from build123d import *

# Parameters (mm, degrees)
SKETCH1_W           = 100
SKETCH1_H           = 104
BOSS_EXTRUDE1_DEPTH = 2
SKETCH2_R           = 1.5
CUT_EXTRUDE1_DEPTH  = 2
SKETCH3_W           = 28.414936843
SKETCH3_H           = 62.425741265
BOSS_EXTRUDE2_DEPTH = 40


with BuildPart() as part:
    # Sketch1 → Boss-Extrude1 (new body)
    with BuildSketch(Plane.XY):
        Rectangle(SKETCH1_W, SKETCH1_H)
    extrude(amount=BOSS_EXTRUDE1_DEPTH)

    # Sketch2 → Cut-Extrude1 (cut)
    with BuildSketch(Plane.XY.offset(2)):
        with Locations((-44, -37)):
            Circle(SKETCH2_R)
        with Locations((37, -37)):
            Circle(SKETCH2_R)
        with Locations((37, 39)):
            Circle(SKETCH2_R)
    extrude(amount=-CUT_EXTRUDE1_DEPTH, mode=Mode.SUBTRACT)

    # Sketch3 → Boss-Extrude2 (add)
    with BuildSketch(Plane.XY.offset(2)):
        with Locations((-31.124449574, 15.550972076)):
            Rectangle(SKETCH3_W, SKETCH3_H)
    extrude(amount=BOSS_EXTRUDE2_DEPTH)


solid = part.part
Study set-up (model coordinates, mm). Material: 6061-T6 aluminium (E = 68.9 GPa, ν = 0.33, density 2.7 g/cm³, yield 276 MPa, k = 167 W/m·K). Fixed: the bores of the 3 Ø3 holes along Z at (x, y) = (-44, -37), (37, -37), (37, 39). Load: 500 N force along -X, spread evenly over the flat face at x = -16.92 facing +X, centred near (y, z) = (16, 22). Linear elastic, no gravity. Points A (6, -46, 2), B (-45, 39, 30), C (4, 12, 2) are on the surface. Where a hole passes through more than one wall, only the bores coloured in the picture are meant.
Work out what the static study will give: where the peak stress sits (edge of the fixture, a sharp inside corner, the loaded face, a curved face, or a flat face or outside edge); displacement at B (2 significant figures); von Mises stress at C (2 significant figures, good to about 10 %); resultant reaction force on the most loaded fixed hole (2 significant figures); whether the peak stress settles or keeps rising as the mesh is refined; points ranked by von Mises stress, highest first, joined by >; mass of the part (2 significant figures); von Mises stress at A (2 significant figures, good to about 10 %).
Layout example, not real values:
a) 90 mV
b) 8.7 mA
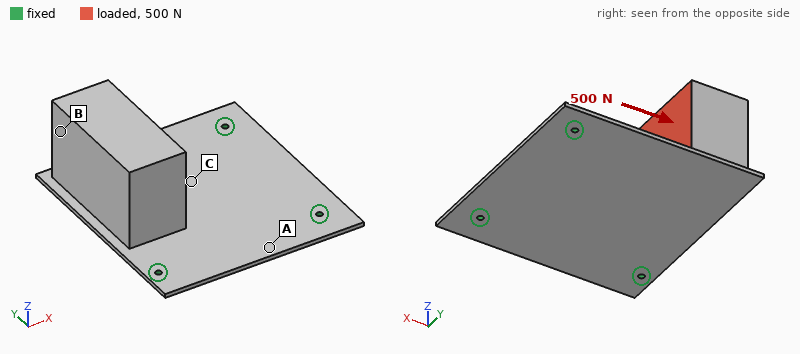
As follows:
a) edge of the fixture
b) 1.3 mm
c) 48 MPa
d) 220 N
e) keeps rising
f) C > A > B
g) 250 g
h) 26 MPa
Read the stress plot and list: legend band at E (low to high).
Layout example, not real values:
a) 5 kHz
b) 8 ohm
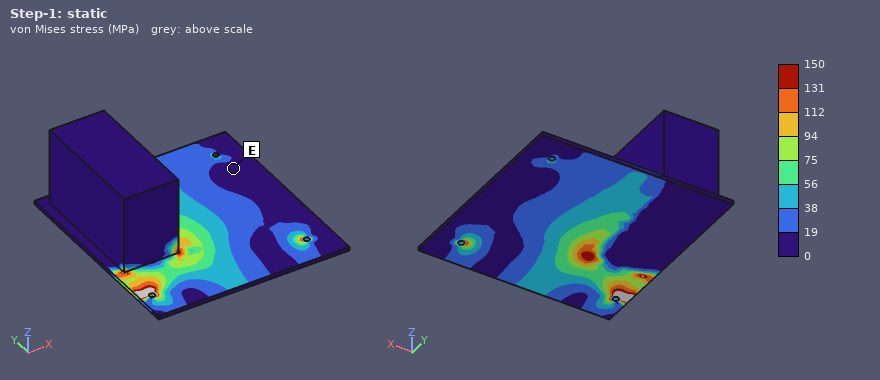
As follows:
a) 0 to 19 MPa
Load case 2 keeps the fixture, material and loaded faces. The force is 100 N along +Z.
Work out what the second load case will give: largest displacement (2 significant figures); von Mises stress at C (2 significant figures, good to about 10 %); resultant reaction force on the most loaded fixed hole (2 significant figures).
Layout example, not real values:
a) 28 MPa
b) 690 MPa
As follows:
a) 0.62 mm
b) 17 MPa
c) 58 N
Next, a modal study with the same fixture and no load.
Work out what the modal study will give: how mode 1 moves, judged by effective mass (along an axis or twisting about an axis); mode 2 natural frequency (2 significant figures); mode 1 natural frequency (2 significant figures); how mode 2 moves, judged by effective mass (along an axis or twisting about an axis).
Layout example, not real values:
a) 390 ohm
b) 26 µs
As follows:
a) along Z
b) 370 Hz
c) 140 Hz
d) along X
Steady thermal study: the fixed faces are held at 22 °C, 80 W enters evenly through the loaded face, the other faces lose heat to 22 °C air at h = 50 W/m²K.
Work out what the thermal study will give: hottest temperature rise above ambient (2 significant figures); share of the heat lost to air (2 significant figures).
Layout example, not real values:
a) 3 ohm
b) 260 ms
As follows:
a) 64 K
b) 59 %
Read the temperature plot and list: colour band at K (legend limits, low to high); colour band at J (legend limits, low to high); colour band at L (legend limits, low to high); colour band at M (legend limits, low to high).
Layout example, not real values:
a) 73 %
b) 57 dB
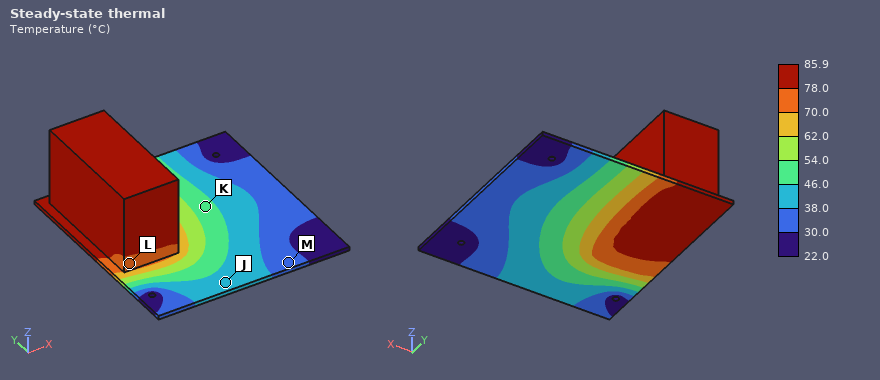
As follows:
a) 46.0 to 54.0 °C
b) 38.0 to 46.0 °C
c) 70.0 to 78.0 °C
d) 30.0 to 38.0 °C
